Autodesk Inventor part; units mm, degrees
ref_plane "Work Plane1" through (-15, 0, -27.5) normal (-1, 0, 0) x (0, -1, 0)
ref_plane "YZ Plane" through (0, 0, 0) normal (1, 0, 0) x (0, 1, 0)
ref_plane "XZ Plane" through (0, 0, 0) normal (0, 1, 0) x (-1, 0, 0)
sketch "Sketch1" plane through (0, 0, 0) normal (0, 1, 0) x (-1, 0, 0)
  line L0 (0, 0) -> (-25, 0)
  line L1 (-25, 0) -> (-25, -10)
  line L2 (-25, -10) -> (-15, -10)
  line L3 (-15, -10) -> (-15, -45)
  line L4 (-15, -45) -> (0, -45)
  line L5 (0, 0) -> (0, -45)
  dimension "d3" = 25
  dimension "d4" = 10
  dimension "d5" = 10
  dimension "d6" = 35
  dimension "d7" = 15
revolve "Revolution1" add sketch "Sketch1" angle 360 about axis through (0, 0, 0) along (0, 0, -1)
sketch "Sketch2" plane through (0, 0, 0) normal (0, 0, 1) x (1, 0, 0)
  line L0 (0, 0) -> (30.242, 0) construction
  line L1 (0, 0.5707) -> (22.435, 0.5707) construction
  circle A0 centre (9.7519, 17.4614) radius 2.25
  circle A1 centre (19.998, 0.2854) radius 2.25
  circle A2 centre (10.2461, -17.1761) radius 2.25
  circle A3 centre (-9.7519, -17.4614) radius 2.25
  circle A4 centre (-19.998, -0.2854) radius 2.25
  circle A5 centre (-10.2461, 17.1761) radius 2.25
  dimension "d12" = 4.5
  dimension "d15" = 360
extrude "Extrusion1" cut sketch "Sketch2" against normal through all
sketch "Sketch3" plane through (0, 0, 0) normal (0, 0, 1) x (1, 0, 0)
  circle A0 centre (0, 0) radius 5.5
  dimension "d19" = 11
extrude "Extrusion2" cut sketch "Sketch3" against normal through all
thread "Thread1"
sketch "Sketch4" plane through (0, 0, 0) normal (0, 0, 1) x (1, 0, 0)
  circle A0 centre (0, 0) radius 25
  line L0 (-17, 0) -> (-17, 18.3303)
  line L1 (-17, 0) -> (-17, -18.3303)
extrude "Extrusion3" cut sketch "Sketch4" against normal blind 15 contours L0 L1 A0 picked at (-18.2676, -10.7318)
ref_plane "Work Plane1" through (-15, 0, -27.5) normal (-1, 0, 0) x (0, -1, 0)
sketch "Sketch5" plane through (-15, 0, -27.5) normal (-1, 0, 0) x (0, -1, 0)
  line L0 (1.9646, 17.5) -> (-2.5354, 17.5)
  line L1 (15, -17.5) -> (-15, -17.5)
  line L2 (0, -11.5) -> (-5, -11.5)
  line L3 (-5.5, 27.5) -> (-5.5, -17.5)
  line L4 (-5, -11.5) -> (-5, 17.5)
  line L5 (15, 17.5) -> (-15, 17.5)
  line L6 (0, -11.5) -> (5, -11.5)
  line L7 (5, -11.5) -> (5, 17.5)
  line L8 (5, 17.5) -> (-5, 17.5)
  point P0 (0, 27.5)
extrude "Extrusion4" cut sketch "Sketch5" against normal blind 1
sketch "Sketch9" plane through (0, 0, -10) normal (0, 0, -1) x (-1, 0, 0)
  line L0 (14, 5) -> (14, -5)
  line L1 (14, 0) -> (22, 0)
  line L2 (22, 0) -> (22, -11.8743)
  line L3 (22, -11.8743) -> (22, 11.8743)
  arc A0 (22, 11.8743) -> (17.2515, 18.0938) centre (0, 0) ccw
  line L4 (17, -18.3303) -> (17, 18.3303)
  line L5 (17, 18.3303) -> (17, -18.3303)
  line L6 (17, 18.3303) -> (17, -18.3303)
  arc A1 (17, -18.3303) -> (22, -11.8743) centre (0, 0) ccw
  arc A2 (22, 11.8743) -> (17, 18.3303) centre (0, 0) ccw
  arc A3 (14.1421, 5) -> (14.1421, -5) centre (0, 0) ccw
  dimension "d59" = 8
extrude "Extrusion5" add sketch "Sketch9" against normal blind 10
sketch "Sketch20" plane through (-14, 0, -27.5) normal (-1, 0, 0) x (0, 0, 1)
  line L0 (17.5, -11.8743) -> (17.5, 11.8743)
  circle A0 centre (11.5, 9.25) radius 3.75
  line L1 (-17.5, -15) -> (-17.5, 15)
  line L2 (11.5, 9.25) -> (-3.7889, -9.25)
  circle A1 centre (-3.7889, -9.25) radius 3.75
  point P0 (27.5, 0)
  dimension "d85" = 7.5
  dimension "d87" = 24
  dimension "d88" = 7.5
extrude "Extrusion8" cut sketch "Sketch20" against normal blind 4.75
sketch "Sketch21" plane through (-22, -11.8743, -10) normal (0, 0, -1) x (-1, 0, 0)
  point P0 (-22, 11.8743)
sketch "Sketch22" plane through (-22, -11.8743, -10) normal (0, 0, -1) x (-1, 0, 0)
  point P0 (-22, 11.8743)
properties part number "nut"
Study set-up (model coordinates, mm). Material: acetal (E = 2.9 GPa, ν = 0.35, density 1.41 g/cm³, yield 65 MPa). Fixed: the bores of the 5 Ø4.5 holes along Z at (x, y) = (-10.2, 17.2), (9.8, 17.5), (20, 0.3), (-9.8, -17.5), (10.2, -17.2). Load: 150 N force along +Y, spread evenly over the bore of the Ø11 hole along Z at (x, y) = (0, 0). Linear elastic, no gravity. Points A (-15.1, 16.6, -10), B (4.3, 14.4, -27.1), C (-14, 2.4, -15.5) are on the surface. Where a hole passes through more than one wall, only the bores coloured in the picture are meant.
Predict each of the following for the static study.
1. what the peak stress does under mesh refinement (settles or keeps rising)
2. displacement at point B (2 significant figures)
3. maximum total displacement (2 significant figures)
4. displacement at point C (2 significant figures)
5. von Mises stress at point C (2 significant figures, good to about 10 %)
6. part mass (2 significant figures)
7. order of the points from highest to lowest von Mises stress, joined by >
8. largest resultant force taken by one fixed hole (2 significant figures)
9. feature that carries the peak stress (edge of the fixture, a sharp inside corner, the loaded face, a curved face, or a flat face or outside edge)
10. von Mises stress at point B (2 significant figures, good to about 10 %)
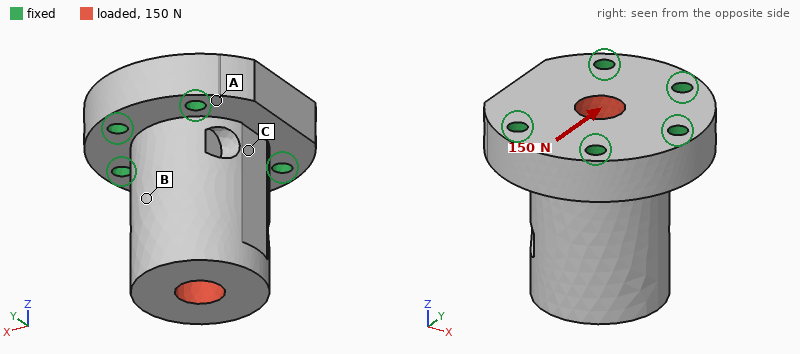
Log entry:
keeps rising
10 µm
18 µm
3.3 µm
0.41 MPa
54 g
C > B > A
56 N
edge of the fixture
0.20 MPa
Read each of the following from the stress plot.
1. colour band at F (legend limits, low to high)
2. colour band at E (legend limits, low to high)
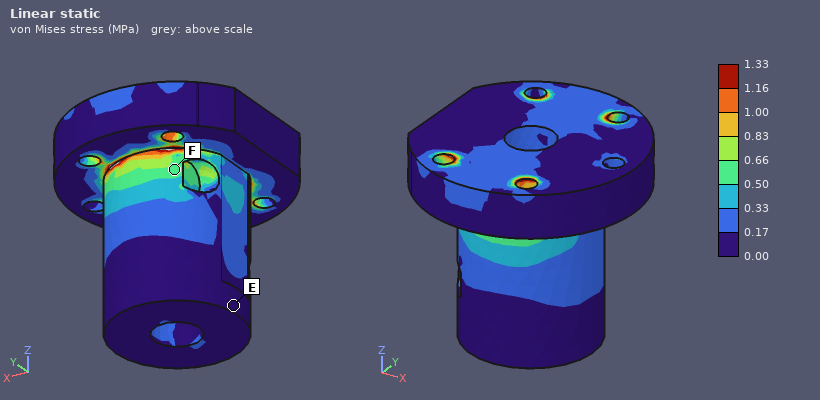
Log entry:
0.50 to 0.66 MPa
0.00 to 0.17 MPa
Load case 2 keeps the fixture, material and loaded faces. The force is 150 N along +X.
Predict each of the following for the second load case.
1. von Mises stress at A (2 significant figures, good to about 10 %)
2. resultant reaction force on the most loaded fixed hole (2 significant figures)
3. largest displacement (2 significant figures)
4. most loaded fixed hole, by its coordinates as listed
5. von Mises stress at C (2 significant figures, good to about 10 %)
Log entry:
0.51 MPa
71 N
23 µm
(20, 0.3)
0.44 MPa
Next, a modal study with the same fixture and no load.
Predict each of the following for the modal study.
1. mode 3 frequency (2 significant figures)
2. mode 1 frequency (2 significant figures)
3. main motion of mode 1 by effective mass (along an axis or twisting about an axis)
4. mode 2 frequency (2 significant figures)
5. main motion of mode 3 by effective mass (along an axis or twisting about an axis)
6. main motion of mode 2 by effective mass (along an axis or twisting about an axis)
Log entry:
5500 Hz
2500 Hz
along X
2800 Hz
twisting about Z
along Y
